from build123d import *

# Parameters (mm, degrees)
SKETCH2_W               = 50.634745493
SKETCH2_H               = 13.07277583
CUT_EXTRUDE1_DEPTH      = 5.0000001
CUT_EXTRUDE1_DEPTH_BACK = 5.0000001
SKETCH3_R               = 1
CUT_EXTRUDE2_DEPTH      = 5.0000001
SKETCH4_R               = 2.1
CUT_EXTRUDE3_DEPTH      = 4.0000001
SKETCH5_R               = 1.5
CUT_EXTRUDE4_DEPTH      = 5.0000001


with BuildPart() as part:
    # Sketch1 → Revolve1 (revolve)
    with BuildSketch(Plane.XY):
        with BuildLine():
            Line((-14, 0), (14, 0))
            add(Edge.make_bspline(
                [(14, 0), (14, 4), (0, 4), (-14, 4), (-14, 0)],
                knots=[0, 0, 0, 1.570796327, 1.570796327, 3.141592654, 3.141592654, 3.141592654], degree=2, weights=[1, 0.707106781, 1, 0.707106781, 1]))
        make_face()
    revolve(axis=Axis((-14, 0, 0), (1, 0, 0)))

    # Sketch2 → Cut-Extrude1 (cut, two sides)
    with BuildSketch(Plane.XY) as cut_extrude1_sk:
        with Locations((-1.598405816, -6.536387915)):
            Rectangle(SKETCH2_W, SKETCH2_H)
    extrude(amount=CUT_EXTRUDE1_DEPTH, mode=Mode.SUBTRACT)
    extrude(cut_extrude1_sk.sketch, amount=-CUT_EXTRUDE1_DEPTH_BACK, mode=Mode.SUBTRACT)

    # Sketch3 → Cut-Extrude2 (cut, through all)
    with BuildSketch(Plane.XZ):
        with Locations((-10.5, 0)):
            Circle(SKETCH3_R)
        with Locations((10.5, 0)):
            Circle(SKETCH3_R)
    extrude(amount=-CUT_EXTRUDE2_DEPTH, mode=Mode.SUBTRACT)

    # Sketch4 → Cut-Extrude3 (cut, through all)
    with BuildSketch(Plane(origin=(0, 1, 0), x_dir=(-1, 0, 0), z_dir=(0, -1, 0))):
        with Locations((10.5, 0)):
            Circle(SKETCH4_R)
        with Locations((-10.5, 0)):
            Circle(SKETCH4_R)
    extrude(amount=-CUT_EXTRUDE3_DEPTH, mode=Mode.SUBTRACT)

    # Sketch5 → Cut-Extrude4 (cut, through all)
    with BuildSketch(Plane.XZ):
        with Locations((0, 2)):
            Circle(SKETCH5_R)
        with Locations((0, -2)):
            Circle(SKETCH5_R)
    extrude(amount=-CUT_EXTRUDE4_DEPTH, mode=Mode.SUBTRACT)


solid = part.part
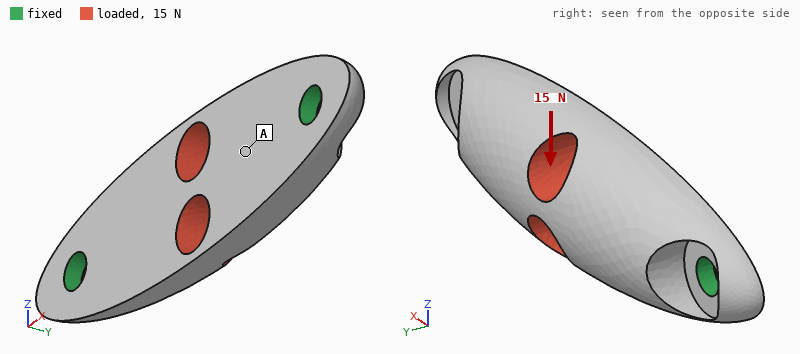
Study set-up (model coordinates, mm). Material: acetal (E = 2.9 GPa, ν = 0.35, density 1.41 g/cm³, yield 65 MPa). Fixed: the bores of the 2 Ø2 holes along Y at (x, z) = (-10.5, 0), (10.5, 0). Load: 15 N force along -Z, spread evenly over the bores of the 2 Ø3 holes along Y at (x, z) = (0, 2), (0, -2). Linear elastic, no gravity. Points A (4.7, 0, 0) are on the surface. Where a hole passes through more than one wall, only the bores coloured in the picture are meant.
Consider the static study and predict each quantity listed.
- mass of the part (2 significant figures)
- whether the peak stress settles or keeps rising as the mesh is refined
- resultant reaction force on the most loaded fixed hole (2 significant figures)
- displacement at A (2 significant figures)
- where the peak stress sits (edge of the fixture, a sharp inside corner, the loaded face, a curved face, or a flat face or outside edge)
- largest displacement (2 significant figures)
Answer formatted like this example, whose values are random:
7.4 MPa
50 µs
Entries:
0.53 g
keeps rising
7.5 N
12 µm
a sharp inside corner
31 µm
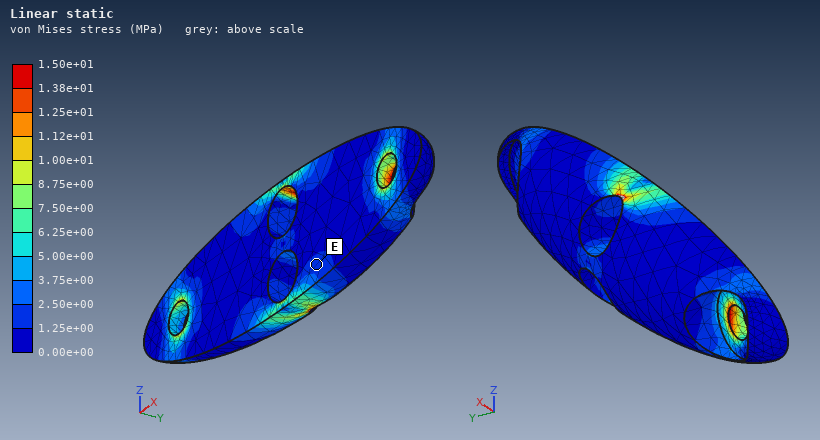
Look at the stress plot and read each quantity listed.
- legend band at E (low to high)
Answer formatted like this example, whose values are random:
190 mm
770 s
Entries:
1.25e+00 to 2.50e+00 MPa
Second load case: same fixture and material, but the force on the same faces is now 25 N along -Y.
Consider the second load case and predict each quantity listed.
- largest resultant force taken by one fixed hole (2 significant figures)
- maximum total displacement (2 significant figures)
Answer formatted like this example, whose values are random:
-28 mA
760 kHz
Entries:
26 N
71 µm
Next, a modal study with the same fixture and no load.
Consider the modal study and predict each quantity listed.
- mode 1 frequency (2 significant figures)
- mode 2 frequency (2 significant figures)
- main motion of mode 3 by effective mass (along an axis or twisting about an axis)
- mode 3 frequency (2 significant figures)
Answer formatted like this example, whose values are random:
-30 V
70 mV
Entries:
6400 Hz
6600 Hz
along Z
9500 Hz
